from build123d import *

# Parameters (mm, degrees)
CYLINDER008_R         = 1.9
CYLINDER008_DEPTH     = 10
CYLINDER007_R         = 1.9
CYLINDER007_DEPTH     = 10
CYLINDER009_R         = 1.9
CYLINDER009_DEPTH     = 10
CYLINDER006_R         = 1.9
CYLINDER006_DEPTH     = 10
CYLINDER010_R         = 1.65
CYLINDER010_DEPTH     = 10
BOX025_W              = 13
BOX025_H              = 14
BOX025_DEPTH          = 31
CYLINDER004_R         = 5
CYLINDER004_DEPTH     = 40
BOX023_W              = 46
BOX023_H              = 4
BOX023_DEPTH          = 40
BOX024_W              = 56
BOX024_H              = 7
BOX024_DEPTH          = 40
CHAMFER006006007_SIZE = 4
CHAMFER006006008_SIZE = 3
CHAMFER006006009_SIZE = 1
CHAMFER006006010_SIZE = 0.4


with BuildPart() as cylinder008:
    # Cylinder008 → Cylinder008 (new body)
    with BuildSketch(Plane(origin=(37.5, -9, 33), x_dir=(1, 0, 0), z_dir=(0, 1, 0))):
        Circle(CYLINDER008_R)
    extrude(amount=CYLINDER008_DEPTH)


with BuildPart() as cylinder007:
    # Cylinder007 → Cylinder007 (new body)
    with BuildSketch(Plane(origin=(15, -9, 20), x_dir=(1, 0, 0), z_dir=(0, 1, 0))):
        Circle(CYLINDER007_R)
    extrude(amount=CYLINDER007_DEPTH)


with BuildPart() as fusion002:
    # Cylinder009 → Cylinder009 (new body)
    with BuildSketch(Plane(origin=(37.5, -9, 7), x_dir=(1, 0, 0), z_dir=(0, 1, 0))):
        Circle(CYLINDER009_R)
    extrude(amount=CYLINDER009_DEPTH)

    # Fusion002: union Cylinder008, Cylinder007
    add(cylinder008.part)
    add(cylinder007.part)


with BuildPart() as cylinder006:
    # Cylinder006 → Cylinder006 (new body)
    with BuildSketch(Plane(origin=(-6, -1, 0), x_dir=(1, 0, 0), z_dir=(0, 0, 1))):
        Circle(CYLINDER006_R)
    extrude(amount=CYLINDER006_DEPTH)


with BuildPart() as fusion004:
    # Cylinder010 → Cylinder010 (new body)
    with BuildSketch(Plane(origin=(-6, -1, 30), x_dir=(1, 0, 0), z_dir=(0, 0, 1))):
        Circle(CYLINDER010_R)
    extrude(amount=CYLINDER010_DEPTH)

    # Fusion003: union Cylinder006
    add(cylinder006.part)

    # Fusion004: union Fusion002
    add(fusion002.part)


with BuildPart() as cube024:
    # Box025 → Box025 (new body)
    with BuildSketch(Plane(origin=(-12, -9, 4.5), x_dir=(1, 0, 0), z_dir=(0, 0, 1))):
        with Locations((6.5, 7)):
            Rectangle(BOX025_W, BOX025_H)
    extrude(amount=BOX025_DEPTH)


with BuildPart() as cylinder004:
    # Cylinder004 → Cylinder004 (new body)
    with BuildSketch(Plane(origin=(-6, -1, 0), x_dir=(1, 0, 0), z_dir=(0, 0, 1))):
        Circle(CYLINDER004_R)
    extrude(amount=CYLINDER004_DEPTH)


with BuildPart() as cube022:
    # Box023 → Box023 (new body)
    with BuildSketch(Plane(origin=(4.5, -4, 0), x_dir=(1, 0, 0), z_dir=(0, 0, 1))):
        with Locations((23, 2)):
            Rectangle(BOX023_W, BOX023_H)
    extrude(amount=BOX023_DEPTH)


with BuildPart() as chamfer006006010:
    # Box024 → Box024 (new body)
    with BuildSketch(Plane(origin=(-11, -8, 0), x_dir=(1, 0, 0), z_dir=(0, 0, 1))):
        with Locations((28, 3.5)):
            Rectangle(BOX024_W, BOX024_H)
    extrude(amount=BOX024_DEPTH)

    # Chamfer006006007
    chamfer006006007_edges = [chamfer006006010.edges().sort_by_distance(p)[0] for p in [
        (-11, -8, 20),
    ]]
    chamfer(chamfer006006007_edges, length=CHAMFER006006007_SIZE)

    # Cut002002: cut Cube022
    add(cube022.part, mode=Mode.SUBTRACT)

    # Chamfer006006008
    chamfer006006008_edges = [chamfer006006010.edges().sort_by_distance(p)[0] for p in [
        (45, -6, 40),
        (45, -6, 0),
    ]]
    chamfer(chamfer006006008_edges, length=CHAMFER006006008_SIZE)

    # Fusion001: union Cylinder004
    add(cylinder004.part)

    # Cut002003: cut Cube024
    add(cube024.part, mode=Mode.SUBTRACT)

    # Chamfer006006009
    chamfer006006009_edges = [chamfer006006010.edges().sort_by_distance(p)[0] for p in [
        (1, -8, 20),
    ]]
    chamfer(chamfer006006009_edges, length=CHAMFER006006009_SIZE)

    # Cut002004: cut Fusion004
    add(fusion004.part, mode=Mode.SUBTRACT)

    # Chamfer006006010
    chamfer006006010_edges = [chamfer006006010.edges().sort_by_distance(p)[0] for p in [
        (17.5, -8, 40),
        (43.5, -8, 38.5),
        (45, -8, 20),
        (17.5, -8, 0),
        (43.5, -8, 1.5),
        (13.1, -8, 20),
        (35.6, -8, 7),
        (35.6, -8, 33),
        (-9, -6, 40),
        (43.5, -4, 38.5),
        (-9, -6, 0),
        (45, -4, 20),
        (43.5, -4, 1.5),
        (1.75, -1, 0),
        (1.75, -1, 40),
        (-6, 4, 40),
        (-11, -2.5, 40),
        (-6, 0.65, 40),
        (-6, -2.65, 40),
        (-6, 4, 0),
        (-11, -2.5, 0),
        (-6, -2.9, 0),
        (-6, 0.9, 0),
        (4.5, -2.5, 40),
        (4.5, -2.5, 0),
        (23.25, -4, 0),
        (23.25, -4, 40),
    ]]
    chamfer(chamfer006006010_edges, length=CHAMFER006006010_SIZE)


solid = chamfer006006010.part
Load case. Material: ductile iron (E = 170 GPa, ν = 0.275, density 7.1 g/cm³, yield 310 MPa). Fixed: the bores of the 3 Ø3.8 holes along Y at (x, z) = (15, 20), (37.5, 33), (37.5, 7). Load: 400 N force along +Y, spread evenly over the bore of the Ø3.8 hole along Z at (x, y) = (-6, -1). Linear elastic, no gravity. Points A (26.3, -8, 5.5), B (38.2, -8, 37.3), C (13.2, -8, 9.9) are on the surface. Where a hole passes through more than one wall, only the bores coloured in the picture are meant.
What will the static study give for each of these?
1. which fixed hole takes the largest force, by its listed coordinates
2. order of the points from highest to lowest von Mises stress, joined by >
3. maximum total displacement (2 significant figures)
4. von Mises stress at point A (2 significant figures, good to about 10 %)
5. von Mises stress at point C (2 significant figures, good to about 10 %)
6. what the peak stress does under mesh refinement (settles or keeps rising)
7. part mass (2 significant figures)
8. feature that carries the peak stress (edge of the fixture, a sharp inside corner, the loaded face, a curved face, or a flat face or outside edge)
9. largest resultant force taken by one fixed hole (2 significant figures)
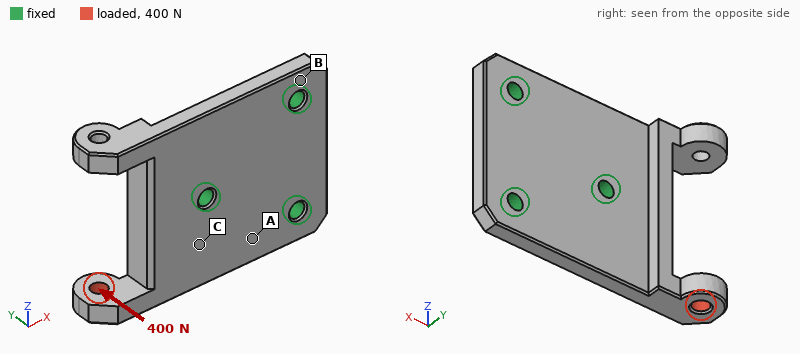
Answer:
(15, 20)
C > A > B
0.17 mm
39 MPa
92 MPa
keeps rising
58 g
edge of the fixture
590 N
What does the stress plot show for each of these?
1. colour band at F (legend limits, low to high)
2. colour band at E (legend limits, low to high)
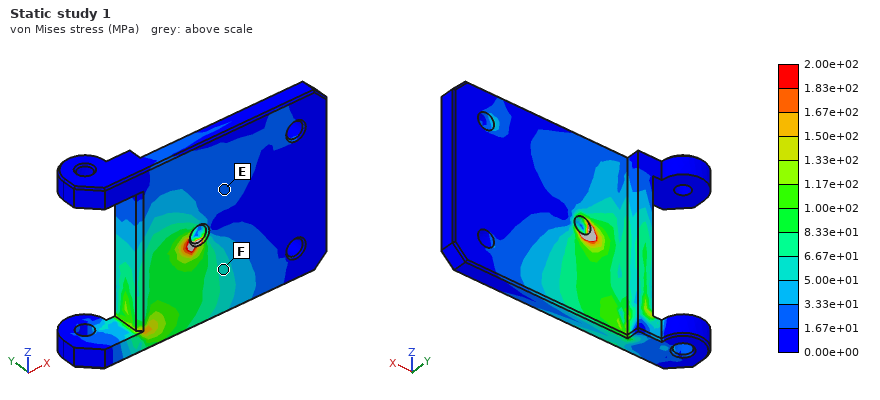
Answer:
5.00e+01 to 6.67e+01 MPa
1.67e+01 to 3.33e+01 MPa
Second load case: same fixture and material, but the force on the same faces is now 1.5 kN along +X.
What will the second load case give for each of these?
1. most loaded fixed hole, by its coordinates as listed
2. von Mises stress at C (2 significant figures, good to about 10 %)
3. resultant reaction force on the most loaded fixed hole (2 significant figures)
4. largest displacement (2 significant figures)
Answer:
(37.5, 7)
66 MPa
1.0 kN
0.18 mm
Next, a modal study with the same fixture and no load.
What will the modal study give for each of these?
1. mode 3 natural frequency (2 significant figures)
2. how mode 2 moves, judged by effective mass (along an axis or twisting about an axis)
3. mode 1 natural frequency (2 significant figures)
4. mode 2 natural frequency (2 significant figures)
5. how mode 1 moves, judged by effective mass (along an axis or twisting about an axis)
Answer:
10 kHz
along Y
4000 Hz
4500 Hz
twisting about X
